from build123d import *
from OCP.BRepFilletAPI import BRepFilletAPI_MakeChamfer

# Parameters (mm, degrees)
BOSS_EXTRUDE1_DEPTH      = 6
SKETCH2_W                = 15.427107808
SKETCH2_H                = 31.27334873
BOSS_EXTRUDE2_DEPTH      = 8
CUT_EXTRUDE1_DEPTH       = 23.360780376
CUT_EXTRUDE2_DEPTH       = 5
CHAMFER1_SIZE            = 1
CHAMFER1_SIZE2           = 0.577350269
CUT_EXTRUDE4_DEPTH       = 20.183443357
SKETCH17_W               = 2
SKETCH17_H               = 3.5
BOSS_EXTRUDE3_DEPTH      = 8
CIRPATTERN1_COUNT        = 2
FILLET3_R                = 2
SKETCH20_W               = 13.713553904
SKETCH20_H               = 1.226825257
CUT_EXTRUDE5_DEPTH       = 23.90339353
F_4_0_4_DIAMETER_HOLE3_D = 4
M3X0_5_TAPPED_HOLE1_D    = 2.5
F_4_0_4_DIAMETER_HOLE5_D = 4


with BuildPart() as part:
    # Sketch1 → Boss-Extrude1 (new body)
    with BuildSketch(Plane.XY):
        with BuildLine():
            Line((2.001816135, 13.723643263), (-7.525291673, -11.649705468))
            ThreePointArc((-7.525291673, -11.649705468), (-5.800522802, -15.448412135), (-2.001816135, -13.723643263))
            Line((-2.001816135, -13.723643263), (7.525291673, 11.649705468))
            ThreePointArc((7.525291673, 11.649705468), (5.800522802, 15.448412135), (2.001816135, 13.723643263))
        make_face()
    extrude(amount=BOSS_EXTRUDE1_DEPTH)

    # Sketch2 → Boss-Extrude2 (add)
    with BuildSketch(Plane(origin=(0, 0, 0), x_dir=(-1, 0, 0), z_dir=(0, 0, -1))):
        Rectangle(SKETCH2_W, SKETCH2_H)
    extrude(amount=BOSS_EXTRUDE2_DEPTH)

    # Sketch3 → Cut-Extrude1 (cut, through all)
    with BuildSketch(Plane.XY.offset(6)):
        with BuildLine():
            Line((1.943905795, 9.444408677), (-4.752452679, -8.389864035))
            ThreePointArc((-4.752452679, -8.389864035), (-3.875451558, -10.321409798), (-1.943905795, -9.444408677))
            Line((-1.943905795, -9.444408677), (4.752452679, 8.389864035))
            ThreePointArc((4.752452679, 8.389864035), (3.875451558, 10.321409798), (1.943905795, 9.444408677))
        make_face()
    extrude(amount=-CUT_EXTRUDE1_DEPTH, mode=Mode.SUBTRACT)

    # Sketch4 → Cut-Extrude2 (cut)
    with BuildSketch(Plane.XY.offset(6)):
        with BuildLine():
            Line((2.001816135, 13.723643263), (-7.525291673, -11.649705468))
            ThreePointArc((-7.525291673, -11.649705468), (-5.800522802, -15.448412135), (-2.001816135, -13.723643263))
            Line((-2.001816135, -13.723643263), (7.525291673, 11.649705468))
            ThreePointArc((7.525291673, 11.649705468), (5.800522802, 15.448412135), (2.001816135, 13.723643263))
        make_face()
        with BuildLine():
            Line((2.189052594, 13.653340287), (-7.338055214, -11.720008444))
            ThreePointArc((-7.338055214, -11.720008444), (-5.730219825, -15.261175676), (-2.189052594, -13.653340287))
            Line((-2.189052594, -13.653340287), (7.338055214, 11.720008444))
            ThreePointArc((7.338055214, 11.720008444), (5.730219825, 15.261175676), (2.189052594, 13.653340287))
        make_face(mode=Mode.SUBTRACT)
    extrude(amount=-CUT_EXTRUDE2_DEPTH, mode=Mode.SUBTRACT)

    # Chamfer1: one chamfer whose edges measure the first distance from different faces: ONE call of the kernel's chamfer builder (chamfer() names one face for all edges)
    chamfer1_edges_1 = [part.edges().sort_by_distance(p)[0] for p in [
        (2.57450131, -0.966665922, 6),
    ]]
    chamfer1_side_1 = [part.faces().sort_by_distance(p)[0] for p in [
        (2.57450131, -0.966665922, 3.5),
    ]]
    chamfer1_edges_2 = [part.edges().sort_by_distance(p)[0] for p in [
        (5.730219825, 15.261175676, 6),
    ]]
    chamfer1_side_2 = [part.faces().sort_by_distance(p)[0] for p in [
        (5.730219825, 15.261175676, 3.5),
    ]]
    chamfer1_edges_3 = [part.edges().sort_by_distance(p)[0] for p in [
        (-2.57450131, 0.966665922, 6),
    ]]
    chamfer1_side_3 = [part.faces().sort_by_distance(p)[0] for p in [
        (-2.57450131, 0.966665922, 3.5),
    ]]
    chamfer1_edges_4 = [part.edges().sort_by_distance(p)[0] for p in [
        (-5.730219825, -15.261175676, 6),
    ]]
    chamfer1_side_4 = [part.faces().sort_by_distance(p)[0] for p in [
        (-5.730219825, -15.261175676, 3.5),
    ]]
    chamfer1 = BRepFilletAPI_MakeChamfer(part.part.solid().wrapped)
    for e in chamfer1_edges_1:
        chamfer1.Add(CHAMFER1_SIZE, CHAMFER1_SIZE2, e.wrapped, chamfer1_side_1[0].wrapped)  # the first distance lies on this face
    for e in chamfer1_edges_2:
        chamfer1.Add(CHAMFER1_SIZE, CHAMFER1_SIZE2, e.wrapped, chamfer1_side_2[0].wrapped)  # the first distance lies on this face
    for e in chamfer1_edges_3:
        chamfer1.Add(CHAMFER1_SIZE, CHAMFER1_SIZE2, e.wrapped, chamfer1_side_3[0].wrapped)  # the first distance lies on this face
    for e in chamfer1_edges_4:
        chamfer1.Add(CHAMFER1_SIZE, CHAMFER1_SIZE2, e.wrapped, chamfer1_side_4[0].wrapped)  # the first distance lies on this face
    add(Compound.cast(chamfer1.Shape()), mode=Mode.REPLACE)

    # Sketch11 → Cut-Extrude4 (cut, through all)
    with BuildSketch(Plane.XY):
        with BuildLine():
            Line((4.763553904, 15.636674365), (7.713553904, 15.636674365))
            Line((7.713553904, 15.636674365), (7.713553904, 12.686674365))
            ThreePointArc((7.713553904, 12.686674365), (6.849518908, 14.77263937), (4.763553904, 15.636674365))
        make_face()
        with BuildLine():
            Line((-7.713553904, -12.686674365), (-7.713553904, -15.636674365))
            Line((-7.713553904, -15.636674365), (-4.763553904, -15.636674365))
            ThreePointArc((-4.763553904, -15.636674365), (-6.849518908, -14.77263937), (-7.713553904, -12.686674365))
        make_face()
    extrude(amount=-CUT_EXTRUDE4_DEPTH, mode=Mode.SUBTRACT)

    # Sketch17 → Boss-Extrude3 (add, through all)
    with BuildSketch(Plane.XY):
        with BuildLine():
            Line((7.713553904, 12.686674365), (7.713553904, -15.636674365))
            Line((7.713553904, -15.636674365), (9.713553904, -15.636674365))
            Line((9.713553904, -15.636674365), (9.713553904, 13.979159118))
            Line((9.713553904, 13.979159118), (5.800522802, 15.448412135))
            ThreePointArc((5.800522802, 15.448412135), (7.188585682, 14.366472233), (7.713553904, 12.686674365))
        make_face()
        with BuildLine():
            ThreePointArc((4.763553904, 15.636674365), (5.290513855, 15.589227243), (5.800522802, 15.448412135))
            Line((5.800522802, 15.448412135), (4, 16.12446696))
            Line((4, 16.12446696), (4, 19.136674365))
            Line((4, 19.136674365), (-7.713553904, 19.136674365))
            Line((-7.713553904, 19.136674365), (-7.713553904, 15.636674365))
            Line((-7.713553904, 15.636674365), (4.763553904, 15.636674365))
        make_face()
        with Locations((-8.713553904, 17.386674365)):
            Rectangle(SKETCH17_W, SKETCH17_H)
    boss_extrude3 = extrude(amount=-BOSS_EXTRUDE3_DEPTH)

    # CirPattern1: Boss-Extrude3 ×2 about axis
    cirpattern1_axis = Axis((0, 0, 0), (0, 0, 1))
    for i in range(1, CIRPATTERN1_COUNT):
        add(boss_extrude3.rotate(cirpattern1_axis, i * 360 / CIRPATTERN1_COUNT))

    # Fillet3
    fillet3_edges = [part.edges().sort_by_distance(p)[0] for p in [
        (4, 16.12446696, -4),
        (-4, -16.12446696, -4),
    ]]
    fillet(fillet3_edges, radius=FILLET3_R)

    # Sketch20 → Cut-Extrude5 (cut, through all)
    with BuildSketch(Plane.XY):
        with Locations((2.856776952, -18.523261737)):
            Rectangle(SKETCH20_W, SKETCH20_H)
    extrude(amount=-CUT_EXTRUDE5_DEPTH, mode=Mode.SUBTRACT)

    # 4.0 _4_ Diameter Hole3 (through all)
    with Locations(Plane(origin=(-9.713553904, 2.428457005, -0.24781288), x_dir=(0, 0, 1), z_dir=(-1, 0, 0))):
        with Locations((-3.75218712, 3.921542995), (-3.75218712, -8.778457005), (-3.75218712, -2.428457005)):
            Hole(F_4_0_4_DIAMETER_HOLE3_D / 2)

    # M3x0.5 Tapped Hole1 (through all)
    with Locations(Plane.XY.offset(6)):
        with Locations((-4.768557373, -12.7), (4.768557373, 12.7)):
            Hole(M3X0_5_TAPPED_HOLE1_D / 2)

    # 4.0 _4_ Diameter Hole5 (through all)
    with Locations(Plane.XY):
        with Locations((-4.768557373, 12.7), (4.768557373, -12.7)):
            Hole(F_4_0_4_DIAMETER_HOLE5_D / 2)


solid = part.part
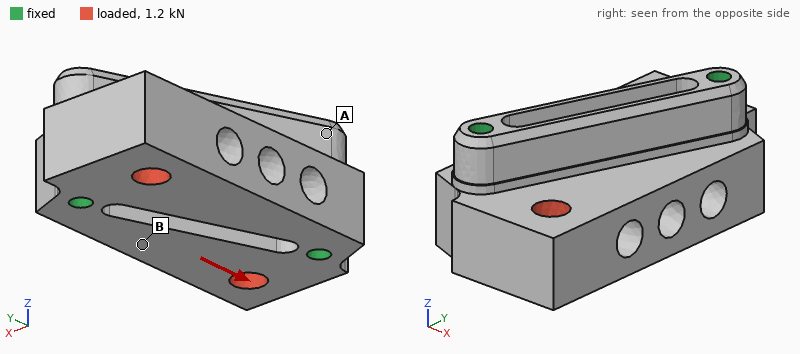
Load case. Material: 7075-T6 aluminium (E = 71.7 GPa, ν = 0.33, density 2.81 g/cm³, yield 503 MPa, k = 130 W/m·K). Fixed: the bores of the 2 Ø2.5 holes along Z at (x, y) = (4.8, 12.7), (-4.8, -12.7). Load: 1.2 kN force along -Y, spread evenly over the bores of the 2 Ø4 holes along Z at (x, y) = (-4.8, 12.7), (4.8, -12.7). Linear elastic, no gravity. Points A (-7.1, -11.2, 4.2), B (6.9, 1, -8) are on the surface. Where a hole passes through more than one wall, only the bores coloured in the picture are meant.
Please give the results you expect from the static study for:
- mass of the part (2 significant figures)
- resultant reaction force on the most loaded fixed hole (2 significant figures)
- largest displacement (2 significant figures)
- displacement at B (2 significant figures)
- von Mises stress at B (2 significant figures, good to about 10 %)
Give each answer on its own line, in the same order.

13 g
600 N
5.4 µm
2.7 µm
12 MPa
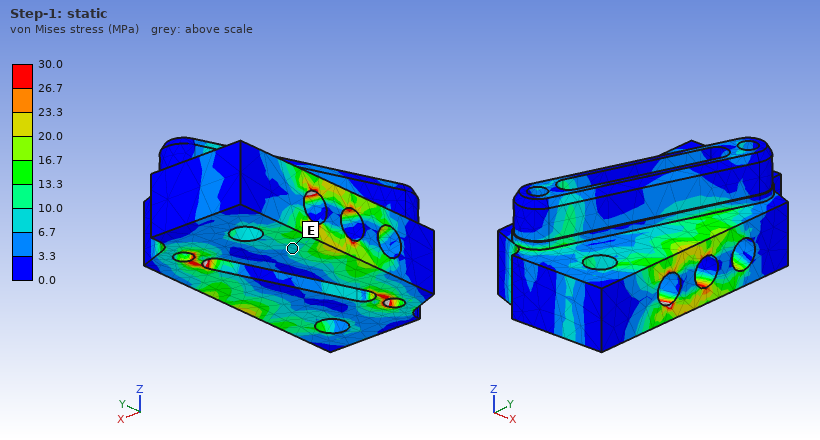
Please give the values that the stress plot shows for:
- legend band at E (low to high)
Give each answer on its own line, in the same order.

6.7 to 10.0 MPa
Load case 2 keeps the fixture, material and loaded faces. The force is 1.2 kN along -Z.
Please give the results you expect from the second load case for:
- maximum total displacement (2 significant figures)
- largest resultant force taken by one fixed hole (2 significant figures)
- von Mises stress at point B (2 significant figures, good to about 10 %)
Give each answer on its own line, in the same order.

14 µm
600 N
12 MPa
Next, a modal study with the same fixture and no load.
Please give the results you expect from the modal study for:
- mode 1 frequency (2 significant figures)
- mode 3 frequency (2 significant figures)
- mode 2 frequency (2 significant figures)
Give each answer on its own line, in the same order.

23 kHz
27 kHz
24 kHz
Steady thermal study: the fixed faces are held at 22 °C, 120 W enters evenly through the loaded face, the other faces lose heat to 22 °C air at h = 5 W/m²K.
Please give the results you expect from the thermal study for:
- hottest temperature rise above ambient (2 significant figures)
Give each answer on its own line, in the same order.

59 K
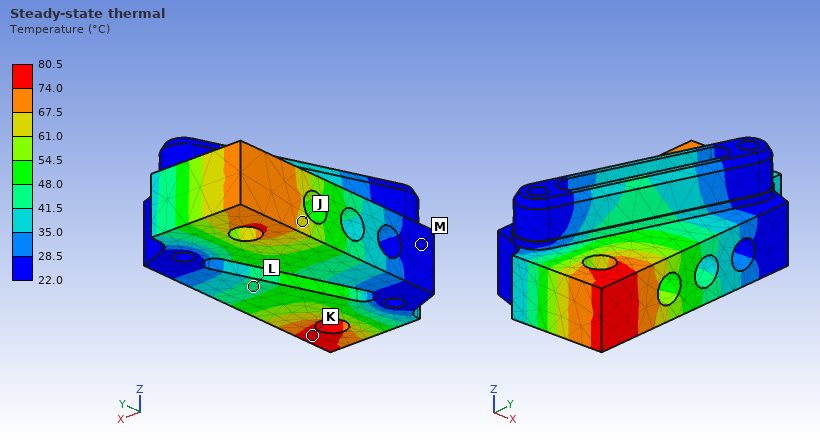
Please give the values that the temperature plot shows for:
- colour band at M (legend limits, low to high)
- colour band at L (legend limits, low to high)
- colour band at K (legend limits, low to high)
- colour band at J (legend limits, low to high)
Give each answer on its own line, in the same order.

22.0 to 28.5 °C
41.5 to 48.0 °C
74.0 to 80.5 °C
61.0 to 67.5 °C
